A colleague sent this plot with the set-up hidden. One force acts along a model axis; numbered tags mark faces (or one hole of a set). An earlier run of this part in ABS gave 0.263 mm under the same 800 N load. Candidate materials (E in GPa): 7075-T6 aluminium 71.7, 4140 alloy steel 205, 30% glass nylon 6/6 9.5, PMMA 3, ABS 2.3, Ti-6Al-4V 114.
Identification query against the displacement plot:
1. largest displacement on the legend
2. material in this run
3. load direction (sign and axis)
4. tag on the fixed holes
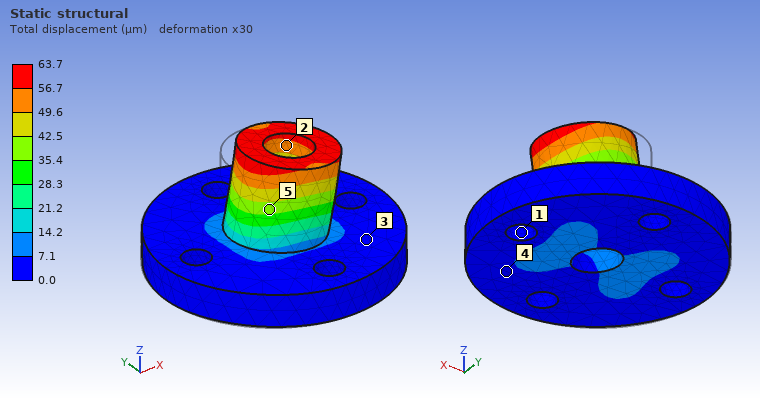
63.7 µm
30% glass nylon 6/6
+X
1
